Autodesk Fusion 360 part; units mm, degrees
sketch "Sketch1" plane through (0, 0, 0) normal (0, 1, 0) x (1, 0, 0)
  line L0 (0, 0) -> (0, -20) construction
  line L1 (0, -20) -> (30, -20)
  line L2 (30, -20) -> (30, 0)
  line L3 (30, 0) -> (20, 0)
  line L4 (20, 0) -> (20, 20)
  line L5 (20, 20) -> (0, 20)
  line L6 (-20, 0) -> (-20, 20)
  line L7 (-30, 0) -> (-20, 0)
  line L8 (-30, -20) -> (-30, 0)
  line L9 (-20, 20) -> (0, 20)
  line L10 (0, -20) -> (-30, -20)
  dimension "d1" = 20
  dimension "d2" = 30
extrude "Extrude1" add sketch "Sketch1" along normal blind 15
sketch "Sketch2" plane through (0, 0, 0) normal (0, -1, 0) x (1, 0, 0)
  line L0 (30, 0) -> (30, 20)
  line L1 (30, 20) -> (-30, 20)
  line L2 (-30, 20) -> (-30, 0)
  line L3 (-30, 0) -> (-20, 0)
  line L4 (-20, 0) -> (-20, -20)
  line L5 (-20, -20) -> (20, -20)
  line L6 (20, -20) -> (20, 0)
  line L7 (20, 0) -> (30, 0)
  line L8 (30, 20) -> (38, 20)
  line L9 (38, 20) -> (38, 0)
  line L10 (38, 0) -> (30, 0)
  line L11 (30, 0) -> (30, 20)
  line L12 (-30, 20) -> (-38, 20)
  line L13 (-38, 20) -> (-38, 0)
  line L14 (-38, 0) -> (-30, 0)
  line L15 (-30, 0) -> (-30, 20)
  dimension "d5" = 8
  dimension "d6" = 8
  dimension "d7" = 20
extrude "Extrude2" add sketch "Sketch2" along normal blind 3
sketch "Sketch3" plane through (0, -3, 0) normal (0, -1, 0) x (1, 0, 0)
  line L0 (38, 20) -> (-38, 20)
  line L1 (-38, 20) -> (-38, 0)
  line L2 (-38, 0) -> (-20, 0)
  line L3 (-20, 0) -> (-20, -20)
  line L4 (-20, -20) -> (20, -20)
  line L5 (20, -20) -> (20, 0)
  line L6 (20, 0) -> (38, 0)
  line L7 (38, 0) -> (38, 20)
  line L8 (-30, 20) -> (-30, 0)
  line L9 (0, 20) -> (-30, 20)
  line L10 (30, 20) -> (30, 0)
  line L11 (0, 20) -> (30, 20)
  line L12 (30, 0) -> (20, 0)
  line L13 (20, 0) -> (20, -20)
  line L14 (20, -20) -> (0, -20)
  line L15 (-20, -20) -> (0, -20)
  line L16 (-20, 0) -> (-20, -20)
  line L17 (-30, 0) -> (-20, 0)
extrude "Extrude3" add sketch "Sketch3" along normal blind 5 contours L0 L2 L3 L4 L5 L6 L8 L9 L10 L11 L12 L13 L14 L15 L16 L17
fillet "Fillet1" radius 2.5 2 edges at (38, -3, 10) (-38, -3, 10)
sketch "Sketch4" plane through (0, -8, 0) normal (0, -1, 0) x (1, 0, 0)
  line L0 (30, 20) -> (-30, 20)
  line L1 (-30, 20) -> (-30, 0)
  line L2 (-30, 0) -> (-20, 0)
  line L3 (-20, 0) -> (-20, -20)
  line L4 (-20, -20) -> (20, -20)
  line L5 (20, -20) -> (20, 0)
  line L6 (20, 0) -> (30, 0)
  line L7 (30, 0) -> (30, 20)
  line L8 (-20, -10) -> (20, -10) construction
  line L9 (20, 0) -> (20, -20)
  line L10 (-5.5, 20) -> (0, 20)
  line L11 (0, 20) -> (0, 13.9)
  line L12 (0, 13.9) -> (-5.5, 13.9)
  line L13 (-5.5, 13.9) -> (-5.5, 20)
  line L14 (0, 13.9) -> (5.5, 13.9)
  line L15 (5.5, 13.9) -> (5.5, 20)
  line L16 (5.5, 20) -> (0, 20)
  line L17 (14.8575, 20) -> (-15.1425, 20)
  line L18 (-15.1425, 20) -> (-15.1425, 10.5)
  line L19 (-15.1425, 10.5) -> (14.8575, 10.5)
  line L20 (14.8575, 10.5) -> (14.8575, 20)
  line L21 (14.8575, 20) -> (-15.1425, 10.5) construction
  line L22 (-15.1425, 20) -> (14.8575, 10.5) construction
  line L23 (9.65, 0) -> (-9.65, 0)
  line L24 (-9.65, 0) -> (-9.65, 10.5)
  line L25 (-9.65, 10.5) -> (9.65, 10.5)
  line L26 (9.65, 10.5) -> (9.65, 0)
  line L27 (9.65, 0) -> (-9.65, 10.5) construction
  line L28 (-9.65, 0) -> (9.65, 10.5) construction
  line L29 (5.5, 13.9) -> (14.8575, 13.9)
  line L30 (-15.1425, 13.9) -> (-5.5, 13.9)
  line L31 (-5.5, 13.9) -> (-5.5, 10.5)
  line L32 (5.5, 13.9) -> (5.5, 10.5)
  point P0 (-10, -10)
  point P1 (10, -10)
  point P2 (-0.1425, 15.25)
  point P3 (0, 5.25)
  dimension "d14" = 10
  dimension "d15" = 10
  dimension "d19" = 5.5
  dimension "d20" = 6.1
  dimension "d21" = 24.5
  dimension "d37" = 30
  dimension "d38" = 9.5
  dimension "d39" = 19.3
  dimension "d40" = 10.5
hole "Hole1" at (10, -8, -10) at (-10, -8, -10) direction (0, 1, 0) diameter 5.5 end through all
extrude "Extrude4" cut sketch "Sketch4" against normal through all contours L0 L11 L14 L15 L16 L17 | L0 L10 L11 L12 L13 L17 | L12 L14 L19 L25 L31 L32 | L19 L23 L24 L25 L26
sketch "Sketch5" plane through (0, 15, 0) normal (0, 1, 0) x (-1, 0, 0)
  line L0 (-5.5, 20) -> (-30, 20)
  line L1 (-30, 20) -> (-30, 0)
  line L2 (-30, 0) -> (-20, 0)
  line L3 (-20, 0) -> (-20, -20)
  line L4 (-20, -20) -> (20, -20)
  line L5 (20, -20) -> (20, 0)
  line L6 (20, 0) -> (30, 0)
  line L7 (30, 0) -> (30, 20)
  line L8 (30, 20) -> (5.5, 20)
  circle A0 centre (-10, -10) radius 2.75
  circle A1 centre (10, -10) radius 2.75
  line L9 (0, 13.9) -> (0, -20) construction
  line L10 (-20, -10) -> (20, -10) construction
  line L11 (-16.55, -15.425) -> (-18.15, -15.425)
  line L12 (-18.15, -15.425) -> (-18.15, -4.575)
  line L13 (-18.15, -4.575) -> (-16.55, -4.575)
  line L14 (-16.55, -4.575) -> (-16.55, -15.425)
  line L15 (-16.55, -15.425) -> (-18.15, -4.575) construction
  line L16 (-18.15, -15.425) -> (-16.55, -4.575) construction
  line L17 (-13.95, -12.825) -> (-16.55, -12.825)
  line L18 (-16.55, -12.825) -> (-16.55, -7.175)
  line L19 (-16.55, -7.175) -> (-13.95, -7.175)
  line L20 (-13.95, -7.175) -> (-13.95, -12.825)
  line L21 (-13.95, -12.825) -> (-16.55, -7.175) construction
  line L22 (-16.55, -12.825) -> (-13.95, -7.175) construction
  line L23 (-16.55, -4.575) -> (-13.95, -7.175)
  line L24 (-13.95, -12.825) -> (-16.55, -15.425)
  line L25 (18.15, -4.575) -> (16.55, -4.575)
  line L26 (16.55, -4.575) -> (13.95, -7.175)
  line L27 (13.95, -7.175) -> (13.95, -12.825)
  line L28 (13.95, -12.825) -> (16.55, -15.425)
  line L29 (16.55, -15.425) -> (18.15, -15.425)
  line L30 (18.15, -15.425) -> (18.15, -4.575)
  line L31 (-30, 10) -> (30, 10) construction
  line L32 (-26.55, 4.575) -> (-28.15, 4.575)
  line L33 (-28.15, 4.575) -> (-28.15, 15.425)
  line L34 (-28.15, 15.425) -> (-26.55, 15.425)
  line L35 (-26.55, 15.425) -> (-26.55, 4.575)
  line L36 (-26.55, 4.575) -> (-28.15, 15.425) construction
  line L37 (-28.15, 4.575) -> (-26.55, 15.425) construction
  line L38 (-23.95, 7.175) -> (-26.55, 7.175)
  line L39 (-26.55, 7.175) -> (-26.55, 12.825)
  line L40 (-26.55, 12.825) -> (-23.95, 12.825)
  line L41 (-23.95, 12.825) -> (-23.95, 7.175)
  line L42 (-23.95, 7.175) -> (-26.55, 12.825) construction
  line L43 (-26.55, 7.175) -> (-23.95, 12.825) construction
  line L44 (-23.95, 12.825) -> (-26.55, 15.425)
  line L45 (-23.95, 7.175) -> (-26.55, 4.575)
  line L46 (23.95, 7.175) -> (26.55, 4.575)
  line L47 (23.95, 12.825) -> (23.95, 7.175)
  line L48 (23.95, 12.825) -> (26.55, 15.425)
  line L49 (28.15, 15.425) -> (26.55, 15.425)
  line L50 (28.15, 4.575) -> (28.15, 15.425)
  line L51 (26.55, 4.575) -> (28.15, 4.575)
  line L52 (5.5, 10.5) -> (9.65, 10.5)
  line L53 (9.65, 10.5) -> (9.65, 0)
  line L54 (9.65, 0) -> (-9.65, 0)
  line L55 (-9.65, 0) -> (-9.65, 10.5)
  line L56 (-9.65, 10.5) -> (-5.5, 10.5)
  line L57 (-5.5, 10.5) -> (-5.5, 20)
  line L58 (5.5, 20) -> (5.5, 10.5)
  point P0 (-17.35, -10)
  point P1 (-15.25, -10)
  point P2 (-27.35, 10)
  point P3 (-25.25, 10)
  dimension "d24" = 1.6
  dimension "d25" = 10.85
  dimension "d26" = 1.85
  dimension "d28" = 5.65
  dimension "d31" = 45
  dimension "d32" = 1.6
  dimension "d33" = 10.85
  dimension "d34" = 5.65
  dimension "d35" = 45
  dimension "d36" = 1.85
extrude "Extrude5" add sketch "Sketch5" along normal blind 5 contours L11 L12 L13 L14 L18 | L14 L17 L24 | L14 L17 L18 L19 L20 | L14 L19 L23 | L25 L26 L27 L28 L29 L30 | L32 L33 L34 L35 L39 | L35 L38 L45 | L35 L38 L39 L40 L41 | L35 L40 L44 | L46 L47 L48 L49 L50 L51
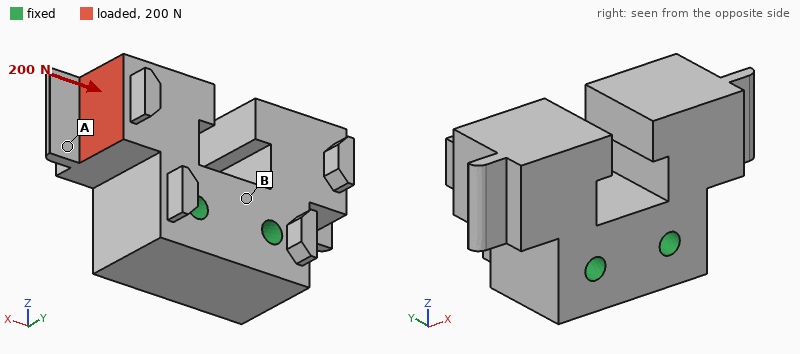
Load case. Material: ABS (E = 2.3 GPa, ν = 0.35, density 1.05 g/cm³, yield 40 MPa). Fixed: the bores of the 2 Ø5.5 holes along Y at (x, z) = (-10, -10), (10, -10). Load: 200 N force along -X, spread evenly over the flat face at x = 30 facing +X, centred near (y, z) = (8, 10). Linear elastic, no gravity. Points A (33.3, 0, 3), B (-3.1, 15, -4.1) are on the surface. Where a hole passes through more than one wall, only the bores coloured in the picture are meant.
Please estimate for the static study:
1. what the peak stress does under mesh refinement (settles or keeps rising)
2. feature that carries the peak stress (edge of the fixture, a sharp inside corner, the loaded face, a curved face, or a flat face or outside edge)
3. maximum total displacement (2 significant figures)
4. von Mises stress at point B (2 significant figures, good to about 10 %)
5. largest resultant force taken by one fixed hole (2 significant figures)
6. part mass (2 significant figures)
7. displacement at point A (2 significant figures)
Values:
keeps rising
a sharp inside corner
0.17 mm
1.1 MPa
160 N
42 g
0.10 mm
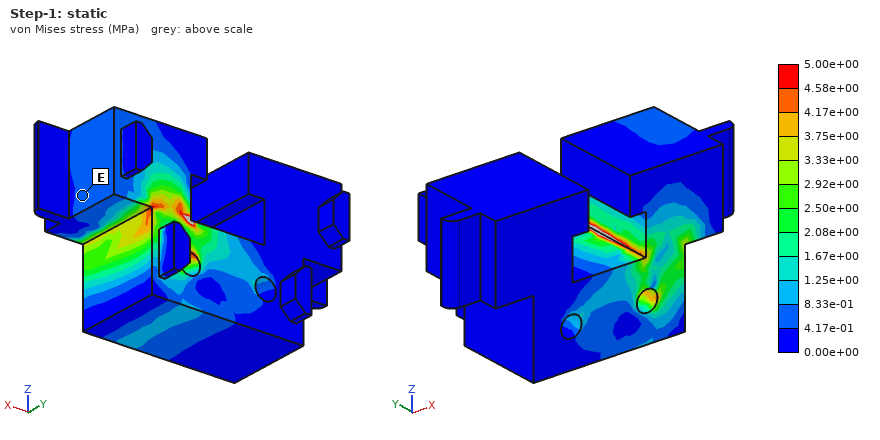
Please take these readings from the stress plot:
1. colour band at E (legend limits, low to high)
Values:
4.17e-01 to 8.33e-01 MPa
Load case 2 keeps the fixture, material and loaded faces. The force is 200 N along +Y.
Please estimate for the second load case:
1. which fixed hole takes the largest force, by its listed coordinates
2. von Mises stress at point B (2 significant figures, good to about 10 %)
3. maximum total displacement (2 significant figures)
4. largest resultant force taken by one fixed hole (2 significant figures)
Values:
(10, -10)
0.82 MPa
0.12 mm
230 N
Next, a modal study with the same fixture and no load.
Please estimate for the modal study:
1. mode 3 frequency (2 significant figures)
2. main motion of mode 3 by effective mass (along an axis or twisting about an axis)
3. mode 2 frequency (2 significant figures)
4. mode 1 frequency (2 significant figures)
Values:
3100 Hz
twisting about Z
1900 Hz
1900 Hz
